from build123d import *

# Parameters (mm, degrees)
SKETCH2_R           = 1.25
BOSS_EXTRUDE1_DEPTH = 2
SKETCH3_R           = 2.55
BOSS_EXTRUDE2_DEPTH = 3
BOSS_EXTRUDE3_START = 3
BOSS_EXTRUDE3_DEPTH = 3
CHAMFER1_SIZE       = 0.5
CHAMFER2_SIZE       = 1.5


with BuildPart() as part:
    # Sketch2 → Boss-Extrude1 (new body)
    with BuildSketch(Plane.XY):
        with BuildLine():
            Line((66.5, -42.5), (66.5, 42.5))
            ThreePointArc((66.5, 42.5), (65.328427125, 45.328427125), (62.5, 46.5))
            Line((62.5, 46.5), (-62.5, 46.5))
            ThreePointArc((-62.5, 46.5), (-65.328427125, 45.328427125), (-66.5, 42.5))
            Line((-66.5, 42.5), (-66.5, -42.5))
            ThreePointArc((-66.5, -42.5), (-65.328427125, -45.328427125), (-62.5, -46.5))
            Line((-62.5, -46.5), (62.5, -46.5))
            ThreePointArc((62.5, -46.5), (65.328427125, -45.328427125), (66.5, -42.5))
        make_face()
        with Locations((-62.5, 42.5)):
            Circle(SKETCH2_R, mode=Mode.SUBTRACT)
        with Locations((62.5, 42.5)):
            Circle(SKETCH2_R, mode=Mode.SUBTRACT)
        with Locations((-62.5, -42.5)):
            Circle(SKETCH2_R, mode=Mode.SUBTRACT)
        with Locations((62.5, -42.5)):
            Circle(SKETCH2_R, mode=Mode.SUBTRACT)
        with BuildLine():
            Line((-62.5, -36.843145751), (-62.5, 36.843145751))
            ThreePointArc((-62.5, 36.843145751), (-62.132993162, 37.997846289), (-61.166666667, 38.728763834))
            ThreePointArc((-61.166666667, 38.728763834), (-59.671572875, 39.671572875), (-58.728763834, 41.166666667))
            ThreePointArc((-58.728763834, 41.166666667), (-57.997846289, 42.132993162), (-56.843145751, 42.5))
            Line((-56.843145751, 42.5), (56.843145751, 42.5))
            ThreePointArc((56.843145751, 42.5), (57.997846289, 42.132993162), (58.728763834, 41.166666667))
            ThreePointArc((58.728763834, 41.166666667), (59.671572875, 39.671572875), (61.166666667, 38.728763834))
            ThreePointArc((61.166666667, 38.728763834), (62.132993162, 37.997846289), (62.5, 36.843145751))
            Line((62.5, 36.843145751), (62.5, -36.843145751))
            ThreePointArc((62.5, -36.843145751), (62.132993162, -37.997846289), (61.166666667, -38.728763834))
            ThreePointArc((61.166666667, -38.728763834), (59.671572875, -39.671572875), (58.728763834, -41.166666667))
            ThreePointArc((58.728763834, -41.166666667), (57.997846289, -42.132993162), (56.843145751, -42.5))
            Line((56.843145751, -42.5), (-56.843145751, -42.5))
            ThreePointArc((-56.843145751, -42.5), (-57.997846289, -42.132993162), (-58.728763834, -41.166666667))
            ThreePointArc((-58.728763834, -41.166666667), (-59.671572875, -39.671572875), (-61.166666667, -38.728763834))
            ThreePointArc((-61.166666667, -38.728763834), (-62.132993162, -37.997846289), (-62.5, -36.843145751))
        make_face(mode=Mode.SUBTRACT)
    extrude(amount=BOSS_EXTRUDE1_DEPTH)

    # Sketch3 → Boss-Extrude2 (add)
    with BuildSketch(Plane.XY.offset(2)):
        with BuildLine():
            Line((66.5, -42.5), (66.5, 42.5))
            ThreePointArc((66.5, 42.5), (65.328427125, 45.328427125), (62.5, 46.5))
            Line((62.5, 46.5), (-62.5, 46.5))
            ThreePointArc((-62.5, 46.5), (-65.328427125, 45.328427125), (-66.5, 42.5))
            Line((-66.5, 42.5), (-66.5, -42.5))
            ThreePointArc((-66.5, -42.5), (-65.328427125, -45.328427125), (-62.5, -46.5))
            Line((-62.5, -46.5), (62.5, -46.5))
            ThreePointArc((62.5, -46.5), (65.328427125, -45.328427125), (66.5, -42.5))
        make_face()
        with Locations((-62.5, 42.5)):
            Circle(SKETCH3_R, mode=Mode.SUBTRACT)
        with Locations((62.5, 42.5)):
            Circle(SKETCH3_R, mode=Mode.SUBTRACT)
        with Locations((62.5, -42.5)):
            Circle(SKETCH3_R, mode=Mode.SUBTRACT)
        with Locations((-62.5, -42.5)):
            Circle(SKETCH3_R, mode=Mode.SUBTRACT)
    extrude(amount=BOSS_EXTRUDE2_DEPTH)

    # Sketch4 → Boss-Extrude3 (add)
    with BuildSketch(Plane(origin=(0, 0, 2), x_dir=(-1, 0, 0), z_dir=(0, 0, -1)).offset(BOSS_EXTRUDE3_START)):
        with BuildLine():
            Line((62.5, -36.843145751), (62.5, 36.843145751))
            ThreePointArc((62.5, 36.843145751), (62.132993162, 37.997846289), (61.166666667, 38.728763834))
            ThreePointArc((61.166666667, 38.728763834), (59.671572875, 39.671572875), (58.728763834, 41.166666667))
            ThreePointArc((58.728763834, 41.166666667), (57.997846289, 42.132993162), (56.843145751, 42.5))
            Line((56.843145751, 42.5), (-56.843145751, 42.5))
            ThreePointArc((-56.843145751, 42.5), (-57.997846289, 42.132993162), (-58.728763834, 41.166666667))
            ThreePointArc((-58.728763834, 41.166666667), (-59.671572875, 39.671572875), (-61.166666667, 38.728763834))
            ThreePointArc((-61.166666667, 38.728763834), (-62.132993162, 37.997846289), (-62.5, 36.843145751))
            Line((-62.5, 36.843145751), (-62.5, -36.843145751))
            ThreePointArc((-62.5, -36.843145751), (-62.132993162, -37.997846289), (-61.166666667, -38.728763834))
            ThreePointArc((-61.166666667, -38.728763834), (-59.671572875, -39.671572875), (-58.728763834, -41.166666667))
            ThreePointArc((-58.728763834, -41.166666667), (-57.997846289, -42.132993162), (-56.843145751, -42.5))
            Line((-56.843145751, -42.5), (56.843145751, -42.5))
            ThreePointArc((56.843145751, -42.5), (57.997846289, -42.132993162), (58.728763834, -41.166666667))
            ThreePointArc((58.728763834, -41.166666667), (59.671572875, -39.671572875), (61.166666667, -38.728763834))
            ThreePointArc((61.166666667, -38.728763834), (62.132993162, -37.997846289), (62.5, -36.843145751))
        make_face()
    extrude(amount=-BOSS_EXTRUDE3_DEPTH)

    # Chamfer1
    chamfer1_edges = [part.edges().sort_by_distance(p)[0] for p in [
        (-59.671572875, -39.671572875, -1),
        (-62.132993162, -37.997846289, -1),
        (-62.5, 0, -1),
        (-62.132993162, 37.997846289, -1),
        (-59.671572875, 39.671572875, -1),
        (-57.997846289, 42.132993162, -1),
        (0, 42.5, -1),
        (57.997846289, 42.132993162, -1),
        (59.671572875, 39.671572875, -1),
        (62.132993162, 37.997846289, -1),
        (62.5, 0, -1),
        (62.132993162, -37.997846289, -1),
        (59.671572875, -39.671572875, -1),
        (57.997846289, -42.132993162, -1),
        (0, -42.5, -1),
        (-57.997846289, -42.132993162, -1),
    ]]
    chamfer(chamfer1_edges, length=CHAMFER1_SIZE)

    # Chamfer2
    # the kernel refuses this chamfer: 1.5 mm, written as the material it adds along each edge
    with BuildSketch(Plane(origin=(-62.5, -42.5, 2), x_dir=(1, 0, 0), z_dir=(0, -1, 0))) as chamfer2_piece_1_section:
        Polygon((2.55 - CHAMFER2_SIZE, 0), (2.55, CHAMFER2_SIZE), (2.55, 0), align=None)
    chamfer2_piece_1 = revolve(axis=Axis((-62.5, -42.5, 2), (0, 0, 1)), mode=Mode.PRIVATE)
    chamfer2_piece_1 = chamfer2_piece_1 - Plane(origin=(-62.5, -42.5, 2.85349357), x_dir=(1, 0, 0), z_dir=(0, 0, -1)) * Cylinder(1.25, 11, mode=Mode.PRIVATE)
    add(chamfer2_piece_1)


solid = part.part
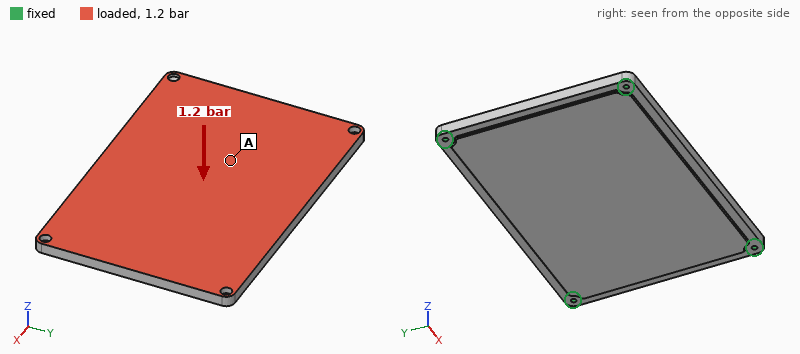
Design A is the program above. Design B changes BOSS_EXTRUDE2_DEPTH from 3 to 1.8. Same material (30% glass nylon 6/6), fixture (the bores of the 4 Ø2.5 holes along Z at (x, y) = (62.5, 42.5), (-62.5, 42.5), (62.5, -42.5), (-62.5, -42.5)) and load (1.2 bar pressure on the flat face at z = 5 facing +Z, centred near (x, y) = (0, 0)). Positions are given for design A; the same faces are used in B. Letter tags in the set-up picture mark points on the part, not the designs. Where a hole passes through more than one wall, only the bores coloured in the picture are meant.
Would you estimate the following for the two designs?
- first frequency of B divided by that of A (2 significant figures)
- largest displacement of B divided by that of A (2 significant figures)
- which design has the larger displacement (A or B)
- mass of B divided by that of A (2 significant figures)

0.84
1.8
B
0.80
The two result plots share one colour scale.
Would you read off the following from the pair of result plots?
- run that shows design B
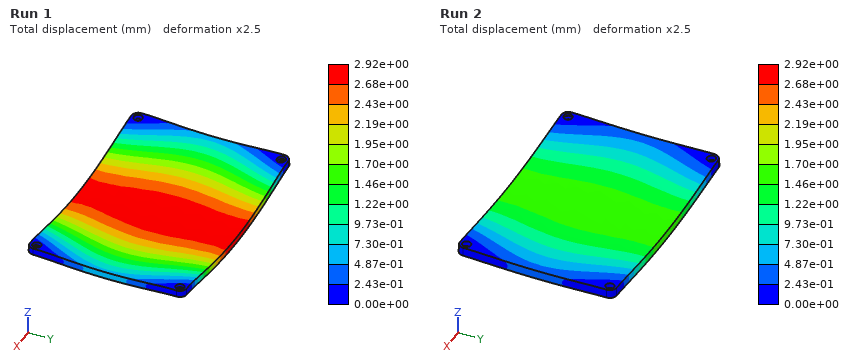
Run 1
